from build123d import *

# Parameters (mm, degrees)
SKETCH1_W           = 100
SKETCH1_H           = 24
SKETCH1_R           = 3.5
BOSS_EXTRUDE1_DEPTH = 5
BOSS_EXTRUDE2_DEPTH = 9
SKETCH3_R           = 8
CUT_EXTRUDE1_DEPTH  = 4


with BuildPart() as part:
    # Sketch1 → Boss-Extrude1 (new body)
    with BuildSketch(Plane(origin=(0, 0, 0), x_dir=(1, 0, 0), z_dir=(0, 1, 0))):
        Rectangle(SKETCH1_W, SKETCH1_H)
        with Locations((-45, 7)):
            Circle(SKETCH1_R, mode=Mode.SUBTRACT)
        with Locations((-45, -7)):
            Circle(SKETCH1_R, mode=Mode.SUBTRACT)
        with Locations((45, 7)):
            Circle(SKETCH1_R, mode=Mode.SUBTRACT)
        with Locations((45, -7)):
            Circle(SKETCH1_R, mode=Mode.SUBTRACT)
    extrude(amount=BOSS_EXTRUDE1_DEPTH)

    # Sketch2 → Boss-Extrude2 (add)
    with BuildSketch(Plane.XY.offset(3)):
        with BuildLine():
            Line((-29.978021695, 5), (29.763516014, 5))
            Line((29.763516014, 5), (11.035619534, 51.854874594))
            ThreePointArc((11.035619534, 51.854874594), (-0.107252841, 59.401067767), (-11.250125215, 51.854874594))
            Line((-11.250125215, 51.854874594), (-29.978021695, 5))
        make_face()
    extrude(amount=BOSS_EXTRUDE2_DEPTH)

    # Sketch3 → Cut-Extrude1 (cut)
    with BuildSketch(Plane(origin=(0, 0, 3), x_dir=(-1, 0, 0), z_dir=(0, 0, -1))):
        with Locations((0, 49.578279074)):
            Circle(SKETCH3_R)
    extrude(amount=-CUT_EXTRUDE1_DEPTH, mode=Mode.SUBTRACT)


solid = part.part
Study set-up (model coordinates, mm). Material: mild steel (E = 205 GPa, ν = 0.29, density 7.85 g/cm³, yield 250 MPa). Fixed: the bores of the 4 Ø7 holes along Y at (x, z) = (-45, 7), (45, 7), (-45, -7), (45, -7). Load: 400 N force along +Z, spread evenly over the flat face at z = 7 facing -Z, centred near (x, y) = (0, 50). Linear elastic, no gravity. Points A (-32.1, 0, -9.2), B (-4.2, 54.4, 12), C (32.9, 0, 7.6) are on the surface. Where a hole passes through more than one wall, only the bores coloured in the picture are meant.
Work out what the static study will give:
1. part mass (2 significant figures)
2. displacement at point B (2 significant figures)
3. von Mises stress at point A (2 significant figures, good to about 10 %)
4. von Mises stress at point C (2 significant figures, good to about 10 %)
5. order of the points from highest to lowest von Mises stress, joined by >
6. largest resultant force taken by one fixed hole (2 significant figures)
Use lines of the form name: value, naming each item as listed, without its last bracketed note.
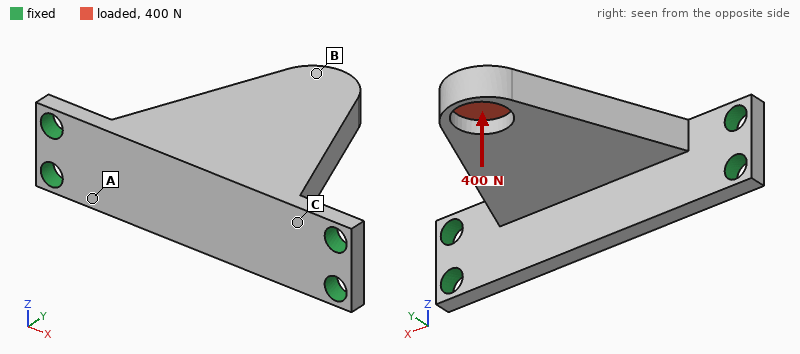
part mass: 230 g
displacement at point B: 0.13 mm
von Mises stress at point A: 34 MPa
von Mises stress at point C: 77 MPa
order of the points from highest to lowest von Mises stress, joined by >: C > A > B
largest resultant force taken by one fixed hole: 610 N
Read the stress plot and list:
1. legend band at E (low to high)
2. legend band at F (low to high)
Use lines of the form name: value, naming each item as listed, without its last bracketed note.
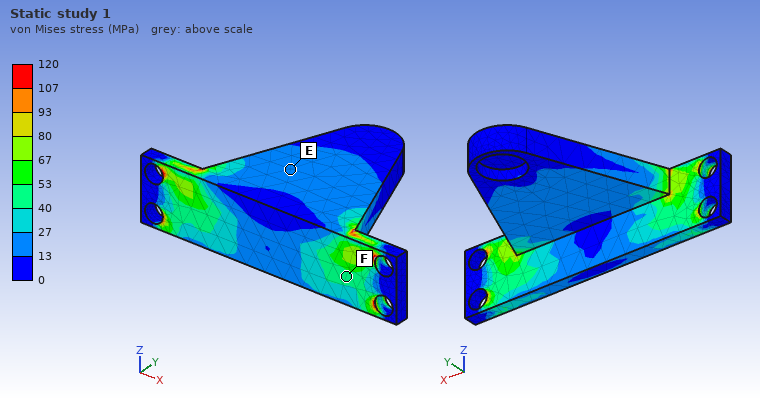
legend band at E: 13 to 27 MPa
legend band at F: 40 to 53 MPa
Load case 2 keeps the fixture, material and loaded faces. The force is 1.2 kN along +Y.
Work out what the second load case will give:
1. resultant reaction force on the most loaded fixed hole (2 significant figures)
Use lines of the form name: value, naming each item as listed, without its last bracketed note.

resultant reaction force on the most loaded fixed hole: 670 N
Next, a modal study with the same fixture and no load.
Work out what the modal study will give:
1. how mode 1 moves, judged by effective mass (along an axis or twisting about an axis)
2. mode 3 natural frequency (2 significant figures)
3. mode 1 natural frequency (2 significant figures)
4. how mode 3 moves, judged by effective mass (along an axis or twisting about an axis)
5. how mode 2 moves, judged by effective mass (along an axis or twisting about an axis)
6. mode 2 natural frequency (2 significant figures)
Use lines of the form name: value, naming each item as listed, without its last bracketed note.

how mode 1 moves, judged by effective mass: along Z
mode 3 natural frequency: 5400 Hz
mode 1 natural frequency: 1400 Hz
how mode 3 moves, judged by effective mass: along X
how mode 2 moves, judged by effective mass: along Y
mode 2 natural frequency: 4300 Hz
